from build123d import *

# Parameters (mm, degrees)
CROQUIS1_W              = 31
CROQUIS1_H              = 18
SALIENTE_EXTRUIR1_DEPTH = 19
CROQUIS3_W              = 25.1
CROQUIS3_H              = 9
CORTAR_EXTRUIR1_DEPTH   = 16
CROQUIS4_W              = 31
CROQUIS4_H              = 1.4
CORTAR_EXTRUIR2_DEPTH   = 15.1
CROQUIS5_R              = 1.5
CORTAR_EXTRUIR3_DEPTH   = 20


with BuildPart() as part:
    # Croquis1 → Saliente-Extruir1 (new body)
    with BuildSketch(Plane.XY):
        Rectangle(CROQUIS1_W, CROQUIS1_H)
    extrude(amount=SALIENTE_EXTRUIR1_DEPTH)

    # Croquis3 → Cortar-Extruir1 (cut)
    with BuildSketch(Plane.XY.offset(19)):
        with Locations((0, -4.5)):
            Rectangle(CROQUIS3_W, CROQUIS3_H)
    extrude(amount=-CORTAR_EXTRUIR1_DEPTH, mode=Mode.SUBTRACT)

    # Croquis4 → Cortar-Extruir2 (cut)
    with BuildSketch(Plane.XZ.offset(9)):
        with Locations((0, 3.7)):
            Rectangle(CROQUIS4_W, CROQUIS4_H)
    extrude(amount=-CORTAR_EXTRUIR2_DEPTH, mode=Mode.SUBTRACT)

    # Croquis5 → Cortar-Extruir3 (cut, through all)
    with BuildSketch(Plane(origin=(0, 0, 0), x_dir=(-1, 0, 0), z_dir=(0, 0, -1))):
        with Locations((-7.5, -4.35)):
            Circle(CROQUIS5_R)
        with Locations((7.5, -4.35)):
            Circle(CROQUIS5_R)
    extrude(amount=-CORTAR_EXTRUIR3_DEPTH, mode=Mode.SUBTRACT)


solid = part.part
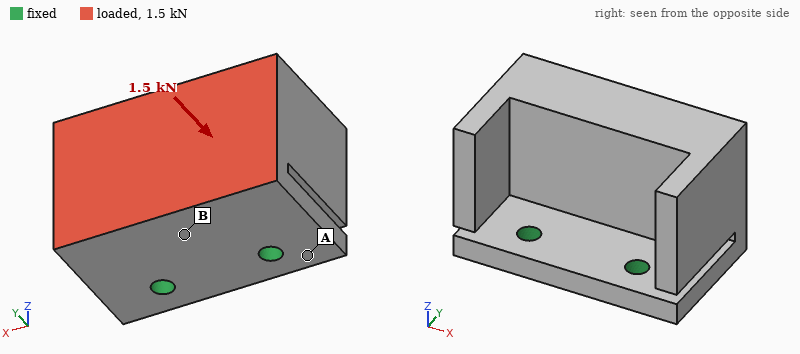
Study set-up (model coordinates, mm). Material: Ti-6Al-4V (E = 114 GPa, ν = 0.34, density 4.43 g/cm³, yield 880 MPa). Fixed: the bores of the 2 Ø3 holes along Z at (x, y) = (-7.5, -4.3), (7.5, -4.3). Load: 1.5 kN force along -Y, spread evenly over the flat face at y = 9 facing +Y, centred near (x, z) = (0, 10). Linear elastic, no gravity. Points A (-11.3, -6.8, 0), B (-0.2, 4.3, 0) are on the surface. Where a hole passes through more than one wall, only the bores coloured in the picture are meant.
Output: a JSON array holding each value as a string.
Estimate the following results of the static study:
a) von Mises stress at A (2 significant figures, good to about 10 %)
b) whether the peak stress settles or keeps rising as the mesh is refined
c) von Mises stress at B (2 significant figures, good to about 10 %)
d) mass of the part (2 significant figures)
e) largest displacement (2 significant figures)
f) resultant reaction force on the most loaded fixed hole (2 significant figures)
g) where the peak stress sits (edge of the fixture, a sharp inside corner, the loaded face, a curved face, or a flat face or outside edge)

["58 MPa", "keeps rising", "220 MPa", "29 g", "0.43 mm", "750 N", "edge of the fixture"]
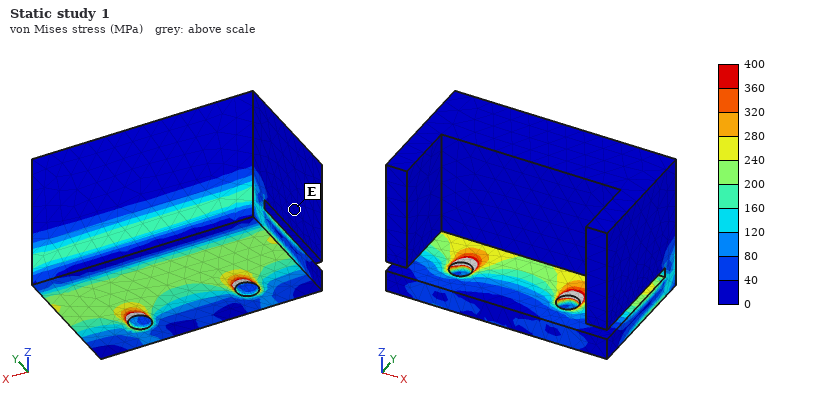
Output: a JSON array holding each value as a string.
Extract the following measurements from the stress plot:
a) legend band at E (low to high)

["0 to 40 MPa"]
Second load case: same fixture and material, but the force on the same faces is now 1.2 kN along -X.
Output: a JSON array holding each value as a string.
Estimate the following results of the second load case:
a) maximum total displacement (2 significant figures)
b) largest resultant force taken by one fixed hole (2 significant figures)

["79 µm", "1.2 kN"]
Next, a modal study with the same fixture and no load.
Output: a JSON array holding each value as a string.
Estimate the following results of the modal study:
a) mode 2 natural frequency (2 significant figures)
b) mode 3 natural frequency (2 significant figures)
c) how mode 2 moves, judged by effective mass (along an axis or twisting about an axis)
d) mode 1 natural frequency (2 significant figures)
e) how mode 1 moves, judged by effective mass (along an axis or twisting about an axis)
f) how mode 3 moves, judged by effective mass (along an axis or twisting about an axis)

["3700 Hz", "5600 Hz", "along X", "2200 Hz", "along Y", "along Z"]
